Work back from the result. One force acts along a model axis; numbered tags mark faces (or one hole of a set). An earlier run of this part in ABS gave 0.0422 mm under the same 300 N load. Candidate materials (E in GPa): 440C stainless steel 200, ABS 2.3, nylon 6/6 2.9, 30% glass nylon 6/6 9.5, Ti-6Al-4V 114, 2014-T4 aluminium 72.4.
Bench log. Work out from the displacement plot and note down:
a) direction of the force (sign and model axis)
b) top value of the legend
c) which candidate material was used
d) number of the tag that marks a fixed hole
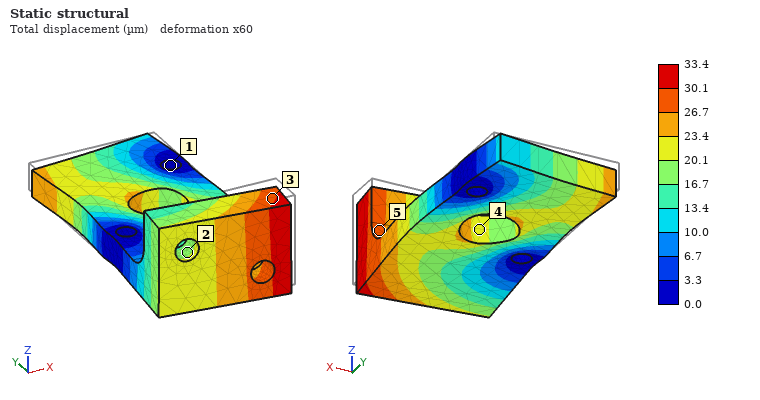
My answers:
-Y
33.4 µm
nylon 6/6
1
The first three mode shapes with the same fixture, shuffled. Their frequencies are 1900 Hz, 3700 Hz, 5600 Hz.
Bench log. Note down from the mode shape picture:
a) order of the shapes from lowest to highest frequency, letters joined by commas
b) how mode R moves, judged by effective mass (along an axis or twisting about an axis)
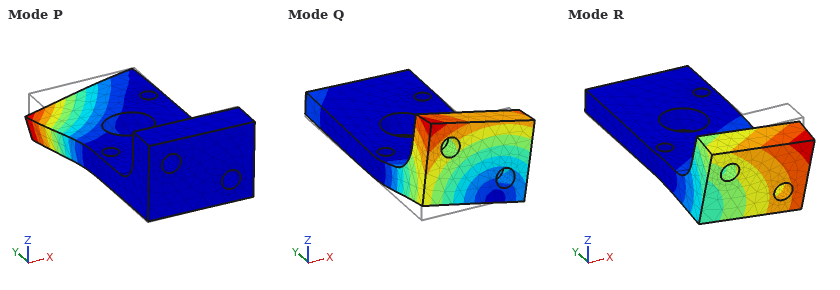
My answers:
R, Q, P
along Z
